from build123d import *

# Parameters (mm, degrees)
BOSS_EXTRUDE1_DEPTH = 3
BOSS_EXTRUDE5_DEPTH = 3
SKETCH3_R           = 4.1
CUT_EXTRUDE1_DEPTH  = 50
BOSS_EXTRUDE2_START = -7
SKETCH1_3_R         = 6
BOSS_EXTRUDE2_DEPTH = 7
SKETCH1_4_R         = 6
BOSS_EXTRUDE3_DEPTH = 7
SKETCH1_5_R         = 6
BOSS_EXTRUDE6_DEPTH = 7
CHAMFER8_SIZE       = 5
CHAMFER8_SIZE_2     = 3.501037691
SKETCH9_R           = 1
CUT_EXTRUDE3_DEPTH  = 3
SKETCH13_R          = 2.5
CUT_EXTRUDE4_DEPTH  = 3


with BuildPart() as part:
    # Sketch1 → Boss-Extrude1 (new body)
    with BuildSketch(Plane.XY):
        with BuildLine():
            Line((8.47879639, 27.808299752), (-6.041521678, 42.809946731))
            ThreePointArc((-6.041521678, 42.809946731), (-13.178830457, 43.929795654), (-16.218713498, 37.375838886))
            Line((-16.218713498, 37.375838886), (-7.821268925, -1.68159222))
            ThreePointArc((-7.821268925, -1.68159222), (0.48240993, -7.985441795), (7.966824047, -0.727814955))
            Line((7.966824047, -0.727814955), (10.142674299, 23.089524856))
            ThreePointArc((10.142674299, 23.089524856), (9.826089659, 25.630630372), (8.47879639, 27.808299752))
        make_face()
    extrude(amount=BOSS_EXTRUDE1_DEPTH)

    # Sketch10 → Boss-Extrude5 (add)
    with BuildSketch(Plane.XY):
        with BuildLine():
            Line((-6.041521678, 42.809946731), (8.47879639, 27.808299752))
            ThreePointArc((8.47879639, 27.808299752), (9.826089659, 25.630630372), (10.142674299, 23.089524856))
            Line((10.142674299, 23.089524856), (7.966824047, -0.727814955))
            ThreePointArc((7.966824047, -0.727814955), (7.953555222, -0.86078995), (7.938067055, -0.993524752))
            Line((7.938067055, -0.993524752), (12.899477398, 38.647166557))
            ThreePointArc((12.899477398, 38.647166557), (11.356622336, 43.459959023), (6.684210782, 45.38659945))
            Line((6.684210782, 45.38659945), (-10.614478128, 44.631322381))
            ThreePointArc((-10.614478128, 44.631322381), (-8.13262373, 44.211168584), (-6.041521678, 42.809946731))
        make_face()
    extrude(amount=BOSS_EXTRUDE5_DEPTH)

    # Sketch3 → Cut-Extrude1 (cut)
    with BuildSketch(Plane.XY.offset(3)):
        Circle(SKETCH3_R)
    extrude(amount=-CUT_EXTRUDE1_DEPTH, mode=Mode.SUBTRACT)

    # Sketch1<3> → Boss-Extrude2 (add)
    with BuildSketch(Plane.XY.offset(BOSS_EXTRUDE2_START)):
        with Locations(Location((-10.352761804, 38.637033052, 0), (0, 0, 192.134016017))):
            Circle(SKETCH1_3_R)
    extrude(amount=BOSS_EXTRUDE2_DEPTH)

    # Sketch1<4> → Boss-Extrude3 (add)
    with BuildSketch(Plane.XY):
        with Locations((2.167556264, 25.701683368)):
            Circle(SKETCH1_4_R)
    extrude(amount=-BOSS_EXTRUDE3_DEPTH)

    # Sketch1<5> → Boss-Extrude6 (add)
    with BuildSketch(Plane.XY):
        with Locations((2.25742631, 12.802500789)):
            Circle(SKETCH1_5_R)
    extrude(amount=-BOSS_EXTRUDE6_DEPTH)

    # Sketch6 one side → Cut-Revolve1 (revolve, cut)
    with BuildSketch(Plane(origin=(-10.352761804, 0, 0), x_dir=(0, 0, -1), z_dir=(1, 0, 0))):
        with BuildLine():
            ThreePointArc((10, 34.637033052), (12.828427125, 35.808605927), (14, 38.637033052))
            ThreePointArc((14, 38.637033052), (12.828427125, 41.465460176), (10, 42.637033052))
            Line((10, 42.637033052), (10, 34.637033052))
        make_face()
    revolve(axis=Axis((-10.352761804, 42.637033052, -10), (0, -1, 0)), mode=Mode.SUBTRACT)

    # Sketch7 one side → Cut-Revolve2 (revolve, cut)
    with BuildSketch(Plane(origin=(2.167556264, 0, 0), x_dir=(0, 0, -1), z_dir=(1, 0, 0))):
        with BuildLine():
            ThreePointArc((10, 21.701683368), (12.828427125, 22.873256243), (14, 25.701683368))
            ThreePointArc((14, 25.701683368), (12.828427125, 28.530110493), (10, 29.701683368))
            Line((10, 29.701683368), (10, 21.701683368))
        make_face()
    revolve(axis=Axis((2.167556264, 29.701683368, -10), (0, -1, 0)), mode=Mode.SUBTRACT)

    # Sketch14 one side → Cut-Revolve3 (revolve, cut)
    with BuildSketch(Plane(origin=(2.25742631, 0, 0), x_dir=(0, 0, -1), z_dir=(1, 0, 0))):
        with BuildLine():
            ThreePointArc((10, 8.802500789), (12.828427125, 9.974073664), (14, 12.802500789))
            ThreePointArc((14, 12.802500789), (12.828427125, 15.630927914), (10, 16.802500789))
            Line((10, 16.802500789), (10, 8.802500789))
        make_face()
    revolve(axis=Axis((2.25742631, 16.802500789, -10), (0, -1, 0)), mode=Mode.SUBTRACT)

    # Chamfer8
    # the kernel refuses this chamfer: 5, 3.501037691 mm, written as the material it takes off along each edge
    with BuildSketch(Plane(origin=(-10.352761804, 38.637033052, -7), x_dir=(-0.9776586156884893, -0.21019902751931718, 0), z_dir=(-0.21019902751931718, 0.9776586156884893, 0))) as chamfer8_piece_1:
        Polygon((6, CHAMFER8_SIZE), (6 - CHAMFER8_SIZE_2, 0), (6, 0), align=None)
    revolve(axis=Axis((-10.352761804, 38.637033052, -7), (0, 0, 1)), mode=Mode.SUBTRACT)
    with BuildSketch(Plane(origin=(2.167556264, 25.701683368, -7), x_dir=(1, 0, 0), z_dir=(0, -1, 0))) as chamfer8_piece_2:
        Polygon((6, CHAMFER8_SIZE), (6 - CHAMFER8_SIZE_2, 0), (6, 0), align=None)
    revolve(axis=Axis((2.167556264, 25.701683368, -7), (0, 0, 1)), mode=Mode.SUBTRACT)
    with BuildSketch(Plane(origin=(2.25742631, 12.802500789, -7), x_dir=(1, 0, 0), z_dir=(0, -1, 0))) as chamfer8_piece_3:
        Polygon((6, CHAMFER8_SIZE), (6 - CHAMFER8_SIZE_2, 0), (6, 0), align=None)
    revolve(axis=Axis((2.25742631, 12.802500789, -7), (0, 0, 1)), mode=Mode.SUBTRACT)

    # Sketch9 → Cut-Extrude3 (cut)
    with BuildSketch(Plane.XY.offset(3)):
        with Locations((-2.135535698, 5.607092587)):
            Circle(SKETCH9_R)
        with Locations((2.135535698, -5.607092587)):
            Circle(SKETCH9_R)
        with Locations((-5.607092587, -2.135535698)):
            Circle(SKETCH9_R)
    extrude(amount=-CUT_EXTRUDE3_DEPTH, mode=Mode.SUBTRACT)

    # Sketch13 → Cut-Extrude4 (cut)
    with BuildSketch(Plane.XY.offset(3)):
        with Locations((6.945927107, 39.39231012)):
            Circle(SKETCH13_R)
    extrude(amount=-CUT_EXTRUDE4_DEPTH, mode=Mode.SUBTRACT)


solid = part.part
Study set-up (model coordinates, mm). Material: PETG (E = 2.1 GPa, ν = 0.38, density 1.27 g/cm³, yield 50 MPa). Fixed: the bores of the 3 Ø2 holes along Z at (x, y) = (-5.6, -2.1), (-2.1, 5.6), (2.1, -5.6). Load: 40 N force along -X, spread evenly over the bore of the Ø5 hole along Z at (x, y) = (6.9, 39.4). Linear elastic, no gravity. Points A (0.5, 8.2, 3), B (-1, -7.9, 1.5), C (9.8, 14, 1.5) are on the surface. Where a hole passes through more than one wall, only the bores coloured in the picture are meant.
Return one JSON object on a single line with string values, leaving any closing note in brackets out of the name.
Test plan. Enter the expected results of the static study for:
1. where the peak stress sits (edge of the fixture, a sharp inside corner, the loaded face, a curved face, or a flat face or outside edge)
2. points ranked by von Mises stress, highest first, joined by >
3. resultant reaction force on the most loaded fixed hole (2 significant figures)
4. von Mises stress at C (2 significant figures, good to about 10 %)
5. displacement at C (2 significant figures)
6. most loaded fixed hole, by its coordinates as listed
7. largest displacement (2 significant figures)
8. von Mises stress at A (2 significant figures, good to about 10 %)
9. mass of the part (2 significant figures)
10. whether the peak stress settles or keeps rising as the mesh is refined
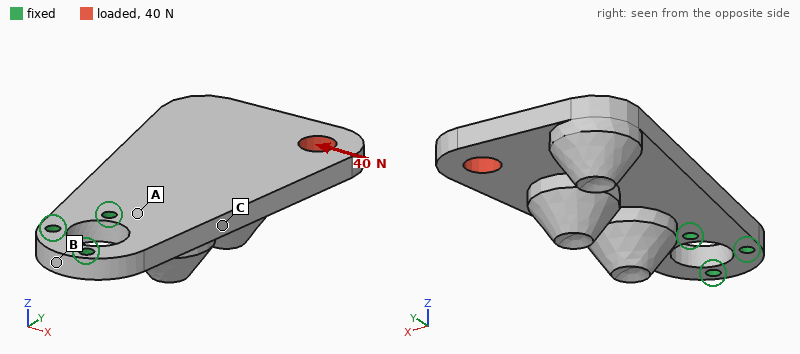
{"where the peak stress sits": "edge of the fixture", "points ranked by von Mises stress, highest first, joined by >": "C > A > B", "resultant reaction force on the most loaded fixed hole": "96 N", "von Mises stress at C": "4.4 MPa", "displacement at C": "0.12 mm", "most loaded fixed hole, by its coordinates as listed": "(-2.1, 5.6)", "largest displacement": "0.42 mm", "von Mises stress at A": "2.5 MPa", "mass of the part": "6.0 g", "whether the peak stress settles or keeps rising as the mesh is refined": "keeps rising"}
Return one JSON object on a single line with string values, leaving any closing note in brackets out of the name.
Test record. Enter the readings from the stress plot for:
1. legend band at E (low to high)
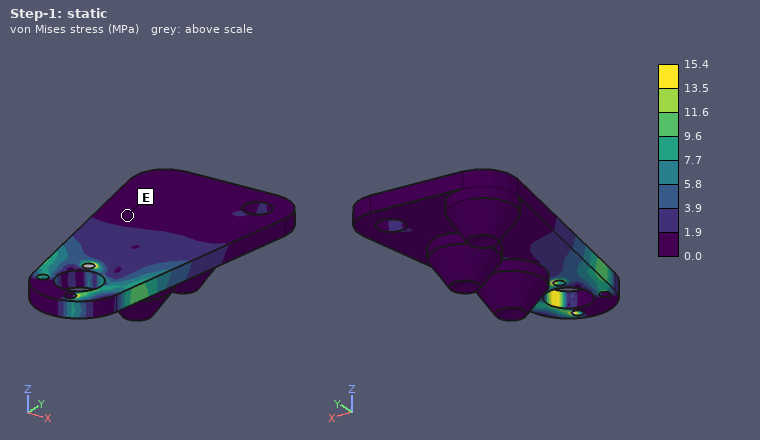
{"legend band at E": "0.0 to 1.9 MPa"}
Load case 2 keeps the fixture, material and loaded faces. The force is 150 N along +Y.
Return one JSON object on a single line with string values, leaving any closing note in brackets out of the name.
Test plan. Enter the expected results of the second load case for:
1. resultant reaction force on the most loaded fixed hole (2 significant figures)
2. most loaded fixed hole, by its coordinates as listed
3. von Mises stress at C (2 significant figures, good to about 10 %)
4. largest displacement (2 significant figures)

{"resultant reaction force on the most loaded fixed hole": "120 N", "most loaded fixed hole, by its coordinates as listed": "(-2.1, 5.6)", "von Mises stress at C": "6.8 MPa", "largest displacement": "0.46 mm"}
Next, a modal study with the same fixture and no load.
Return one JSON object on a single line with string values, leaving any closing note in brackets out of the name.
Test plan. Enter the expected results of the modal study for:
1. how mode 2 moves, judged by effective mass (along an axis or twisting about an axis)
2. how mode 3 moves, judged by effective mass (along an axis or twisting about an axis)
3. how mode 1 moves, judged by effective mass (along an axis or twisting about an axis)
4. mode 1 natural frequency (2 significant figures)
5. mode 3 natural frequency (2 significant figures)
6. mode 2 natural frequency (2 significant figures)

{"how mode 2 moves, judged by effective mass": "along X", "how mode 3 moves, judged by effective mass": "along X", "how mode 1 moves, judged by effective mass": "along Z", "mode 1 natural frequency": "340 Hz", "mode 3 natural frequency": "1100 Hz", "mode 2 natural frequency": "930 Hz"}
